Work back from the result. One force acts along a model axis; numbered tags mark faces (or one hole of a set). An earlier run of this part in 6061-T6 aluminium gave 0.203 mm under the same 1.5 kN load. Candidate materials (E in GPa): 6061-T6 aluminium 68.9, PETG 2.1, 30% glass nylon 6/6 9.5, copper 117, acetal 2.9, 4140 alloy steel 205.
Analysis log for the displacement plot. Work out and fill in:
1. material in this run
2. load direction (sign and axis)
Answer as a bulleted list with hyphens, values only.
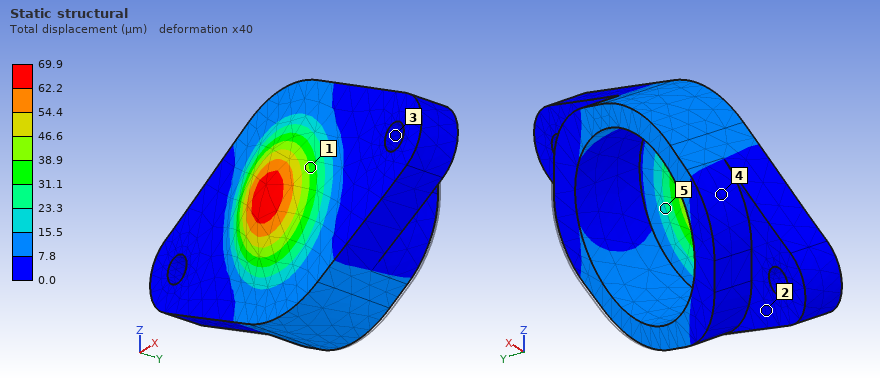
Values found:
- 4140 alloy steel
- -Y
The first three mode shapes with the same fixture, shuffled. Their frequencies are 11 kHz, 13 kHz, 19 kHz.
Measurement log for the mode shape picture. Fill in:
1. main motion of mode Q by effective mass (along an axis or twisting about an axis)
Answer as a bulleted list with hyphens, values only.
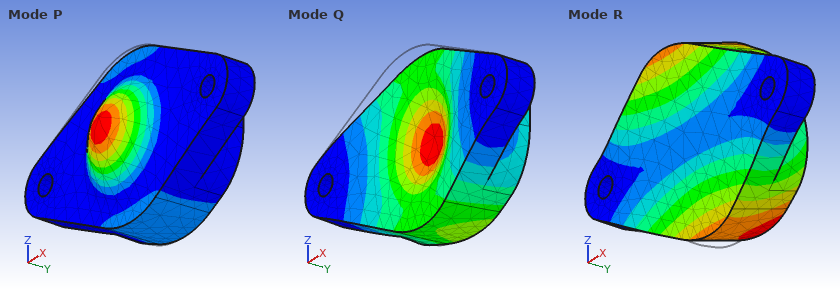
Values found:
- along Y
